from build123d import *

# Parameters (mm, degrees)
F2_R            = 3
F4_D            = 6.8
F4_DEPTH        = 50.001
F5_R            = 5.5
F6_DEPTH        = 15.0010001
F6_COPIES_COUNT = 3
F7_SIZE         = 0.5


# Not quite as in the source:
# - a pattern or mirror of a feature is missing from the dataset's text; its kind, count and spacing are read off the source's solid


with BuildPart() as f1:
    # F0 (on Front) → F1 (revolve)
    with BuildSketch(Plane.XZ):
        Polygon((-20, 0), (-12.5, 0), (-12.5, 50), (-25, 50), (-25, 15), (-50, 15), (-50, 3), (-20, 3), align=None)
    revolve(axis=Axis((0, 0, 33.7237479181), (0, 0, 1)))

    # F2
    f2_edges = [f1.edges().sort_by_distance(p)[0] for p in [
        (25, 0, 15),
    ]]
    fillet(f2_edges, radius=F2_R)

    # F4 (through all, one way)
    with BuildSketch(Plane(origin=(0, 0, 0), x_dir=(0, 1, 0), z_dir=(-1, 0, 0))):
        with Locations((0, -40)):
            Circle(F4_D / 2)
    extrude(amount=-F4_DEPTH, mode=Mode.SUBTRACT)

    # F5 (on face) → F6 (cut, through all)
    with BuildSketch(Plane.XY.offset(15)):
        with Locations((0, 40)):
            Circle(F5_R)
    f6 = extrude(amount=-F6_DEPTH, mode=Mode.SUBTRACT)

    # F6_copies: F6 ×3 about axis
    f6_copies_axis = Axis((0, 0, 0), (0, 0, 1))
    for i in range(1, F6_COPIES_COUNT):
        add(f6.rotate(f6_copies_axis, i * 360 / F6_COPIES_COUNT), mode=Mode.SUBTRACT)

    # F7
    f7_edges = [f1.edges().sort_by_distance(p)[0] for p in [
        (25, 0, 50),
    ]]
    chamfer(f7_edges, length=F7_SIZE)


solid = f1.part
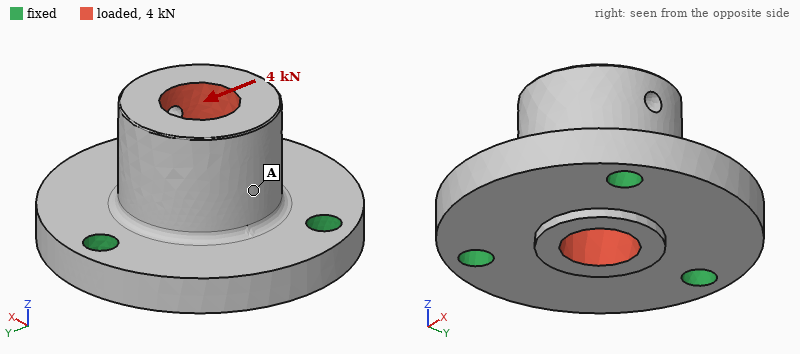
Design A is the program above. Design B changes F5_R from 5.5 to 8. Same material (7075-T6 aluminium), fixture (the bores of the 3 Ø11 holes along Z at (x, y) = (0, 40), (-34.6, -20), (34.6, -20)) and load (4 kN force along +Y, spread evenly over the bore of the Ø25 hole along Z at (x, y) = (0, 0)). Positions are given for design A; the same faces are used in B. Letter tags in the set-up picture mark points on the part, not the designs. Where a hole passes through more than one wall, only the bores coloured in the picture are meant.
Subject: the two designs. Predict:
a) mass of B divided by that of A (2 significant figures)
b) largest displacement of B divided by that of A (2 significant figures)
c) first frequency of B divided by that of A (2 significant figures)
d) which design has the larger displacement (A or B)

0.97
0.84
1.1
A
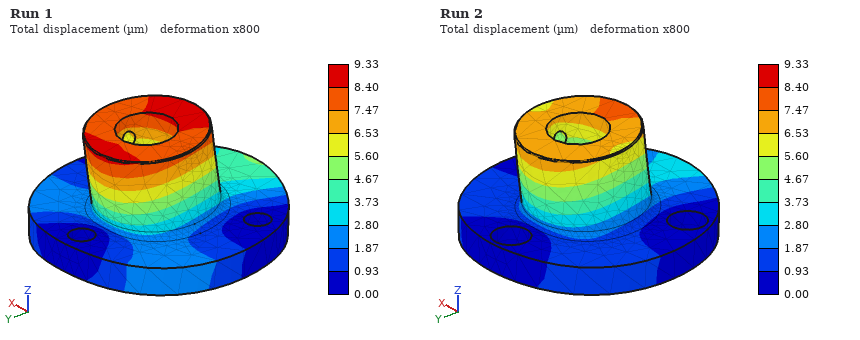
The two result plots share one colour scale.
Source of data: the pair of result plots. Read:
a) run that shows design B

Run 2
